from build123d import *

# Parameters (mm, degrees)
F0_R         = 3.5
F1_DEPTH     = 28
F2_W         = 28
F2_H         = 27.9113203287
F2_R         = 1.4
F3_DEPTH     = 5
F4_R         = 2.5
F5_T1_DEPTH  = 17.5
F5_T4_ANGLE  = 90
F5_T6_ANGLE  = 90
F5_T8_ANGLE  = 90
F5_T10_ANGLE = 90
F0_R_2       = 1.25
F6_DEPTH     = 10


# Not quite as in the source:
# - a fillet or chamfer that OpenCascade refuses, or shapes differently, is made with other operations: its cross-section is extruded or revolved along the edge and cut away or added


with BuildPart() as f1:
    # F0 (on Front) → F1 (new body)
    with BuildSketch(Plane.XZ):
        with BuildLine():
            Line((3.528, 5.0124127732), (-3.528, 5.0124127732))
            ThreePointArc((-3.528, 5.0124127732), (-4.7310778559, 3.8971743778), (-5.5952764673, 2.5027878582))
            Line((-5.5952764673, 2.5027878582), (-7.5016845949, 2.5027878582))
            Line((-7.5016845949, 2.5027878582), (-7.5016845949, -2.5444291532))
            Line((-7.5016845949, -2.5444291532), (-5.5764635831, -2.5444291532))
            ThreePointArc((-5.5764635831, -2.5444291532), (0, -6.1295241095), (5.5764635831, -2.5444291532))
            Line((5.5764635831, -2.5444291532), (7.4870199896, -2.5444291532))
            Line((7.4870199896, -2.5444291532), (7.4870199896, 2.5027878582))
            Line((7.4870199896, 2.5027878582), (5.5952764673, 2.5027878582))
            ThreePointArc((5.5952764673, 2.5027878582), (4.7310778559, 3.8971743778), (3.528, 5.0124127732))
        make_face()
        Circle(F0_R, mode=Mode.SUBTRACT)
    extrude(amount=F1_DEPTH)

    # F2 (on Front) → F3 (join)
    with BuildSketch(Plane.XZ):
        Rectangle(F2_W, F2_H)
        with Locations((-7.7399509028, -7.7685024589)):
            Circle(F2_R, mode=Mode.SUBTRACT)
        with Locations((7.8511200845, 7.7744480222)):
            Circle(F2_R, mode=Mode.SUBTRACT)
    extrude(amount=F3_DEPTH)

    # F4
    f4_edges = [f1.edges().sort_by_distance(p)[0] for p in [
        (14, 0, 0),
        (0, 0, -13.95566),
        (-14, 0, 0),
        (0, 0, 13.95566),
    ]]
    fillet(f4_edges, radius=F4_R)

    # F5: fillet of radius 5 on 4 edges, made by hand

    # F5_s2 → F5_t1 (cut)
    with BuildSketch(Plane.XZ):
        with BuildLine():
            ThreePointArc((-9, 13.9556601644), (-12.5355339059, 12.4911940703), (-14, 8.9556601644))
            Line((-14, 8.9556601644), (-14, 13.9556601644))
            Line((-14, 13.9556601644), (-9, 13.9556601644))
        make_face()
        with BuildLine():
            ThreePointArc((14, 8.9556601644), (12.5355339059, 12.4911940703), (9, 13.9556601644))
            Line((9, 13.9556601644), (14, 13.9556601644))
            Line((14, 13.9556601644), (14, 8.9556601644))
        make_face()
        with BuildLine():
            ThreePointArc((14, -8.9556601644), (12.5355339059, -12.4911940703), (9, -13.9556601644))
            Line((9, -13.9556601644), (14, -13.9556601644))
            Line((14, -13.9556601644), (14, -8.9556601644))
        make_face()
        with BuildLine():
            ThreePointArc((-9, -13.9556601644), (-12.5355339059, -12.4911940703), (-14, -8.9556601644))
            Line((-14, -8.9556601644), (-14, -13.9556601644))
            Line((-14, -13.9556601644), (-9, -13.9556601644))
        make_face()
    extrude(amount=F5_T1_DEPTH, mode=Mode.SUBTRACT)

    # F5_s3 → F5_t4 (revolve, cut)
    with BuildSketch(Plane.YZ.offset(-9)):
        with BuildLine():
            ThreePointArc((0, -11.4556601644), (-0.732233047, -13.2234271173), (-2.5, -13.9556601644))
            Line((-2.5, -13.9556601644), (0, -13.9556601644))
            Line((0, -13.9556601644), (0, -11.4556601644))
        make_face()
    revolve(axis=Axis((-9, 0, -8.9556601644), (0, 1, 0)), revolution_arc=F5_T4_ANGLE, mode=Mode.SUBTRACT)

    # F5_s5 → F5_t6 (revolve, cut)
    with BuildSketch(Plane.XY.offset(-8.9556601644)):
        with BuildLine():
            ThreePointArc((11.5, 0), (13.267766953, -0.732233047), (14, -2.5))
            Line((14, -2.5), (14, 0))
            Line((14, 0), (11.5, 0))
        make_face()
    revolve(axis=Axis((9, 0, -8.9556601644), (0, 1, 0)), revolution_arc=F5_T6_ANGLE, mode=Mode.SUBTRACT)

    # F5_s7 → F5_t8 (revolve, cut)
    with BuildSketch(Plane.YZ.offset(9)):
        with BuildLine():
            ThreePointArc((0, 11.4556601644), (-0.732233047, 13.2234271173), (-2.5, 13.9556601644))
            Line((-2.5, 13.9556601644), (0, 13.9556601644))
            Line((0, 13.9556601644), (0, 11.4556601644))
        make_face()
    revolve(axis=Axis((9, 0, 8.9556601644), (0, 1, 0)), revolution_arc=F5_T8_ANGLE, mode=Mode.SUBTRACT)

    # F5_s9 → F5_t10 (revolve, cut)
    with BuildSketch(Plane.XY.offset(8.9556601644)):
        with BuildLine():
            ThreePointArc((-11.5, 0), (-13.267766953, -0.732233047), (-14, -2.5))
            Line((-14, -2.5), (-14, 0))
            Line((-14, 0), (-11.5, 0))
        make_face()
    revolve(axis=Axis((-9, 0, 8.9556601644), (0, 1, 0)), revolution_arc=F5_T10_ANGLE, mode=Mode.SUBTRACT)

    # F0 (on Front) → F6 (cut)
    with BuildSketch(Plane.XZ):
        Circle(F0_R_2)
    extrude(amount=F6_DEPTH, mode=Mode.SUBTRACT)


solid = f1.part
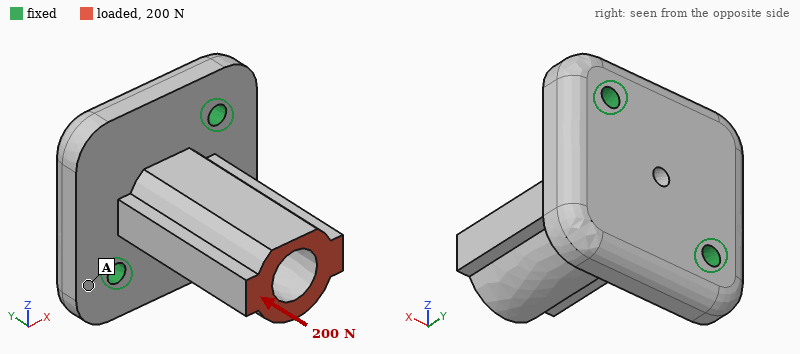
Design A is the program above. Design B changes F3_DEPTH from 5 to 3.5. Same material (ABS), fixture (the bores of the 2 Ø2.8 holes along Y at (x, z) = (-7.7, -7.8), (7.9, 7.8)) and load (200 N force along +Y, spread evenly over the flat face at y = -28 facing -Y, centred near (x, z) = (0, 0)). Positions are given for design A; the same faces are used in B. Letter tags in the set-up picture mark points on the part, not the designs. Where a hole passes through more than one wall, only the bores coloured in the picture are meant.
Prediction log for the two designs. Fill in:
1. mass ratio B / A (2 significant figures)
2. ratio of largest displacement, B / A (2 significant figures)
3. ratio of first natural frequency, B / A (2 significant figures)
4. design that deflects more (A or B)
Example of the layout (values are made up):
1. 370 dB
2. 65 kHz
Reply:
1. 0.83
2. 1.6
3. 0.69
4. B
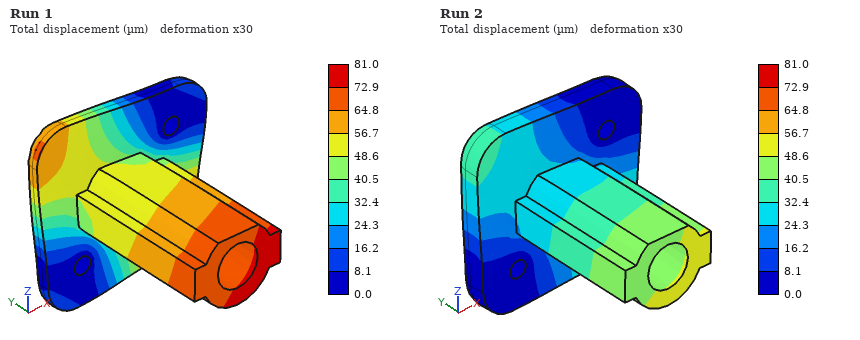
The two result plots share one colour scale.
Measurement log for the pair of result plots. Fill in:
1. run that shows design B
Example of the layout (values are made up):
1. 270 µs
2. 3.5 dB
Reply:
1. Run 1
